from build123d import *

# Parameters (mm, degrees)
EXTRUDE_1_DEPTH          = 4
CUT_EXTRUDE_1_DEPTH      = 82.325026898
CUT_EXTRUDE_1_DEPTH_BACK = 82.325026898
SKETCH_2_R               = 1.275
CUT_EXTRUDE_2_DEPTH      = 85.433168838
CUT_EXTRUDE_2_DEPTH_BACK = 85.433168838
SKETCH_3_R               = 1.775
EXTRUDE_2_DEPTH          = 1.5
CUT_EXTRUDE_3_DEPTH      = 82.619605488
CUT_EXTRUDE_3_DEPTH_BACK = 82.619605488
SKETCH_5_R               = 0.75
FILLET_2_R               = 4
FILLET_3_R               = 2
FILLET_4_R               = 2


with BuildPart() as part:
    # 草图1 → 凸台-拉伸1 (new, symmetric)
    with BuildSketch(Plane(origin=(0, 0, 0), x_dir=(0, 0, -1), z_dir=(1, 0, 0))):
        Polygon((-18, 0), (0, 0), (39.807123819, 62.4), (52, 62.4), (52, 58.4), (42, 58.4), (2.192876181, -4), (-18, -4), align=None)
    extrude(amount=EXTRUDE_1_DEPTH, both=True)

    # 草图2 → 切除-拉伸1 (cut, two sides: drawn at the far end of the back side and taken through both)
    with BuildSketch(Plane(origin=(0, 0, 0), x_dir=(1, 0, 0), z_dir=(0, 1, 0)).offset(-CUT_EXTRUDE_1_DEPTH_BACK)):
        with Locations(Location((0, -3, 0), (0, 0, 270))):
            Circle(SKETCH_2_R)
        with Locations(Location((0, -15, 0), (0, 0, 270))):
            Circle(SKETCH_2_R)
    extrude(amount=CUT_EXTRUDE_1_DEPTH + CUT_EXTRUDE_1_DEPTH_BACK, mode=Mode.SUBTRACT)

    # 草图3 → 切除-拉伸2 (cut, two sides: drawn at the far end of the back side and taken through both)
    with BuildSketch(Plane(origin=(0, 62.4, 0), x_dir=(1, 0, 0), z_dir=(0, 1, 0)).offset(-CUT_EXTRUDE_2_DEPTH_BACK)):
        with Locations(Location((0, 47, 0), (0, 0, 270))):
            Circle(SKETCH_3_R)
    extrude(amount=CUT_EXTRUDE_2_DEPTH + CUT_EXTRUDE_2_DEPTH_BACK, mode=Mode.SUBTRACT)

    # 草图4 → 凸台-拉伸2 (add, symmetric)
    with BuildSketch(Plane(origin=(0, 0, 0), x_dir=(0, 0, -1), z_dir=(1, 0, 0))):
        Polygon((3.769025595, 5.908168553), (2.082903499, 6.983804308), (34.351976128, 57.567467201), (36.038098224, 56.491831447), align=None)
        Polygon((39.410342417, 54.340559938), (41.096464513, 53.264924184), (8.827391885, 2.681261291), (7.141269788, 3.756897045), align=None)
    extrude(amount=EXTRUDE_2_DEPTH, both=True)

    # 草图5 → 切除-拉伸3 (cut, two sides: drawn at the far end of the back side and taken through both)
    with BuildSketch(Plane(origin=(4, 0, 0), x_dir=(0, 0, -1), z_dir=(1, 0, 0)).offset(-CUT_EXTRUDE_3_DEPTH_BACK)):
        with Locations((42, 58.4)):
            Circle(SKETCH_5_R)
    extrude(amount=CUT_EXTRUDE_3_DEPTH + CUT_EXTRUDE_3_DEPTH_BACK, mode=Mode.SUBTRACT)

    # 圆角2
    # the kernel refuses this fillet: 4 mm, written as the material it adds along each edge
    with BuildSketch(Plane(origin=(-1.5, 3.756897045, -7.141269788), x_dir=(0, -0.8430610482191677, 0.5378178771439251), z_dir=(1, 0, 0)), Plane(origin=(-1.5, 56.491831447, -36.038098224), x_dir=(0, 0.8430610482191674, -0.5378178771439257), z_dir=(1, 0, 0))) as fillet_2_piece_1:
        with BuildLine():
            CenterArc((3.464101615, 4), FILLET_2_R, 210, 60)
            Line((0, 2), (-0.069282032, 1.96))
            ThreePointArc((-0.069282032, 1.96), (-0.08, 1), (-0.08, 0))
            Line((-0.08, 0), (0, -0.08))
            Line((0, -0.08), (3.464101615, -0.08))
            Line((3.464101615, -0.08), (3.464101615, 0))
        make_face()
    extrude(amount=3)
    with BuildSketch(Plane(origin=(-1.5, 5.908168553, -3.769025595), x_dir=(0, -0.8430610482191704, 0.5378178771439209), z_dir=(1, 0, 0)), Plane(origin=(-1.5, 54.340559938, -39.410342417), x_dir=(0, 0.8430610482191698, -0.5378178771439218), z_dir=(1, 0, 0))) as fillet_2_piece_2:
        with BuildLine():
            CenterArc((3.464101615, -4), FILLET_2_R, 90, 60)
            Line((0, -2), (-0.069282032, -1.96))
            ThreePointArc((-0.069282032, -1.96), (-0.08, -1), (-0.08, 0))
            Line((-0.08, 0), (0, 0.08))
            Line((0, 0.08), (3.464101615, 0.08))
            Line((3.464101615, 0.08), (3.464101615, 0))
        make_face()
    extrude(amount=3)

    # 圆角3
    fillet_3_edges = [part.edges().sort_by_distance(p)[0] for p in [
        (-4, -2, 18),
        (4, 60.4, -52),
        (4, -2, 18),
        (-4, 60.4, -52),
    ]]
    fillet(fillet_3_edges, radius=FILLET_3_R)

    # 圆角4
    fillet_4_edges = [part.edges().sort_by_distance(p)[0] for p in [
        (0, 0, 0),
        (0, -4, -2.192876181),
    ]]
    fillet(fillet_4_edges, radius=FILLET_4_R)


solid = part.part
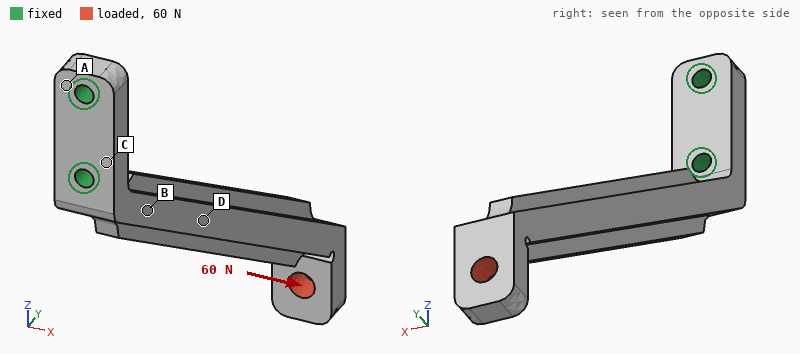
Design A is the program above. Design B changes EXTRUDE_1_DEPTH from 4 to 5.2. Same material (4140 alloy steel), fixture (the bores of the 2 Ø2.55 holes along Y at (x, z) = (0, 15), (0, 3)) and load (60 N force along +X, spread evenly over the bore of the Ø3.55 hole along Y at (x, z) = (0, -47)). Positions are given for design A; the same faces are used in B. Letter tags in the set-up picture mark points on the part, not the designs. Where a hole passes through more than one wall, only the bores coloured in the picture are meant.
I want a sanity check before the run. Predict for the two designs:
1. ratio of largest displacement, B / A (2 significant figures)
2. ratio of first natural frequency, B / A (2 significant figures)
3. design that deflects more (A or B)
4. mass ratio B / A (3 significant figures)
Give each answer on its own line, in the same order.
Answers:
0.54
0.98
A
1.25
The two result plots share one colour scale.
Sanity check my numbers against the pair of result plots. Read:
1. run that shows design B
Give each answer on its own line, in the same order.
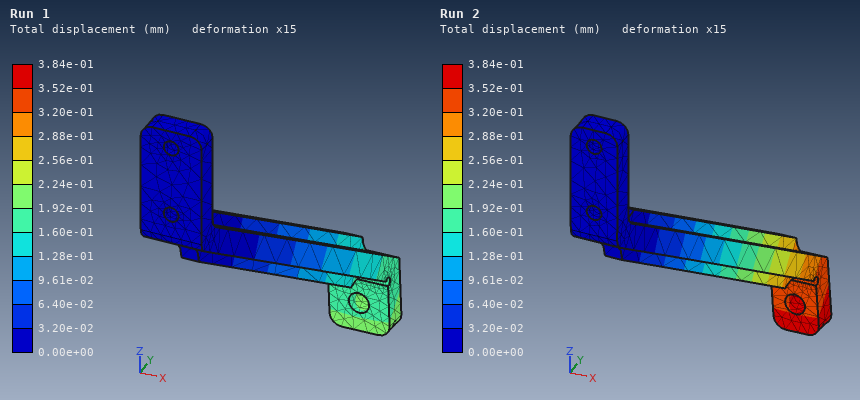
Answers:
Run 1
